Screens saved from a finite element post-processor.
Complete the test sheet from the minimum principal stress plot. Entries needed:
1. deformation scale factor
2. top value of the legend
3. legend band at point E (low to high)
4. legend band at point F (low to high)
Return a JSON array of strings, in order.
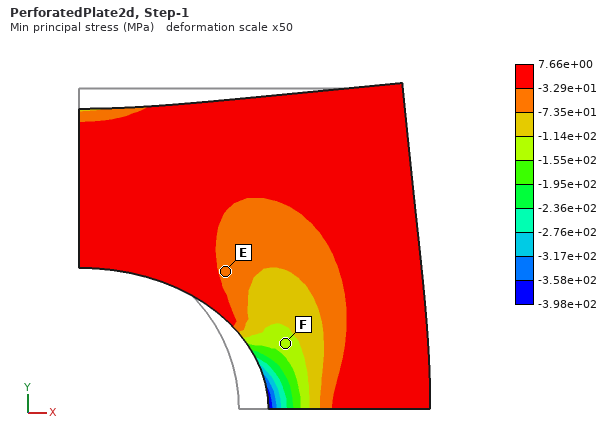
["50", "7.66e+00 MPa", "-7.35e+01 to -3.29e+01 MPa", "-1.55e+02 to -1.14e+02 MPa"]
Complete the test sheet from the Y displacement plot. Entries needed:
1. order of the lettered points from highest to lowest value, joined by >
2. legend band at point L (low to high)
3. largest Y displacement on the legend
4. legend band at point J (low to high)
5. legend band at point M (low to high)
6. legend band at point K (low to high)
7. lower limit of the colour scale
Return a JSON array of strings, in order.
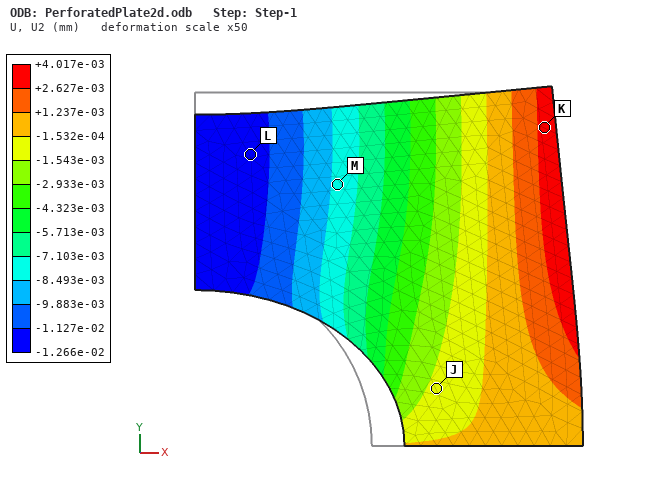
["K > J > M > L", "-1.266e-02 to -1.127e-02 mm", "+4.017e-03 mm", "-1.543e-03 to -1.532e-04 mm", "-8.493e-03 to -7.103e-03 mm", "+2.627e-03 to +4.017e-03 mm", "-1.266e-02 mm"]
